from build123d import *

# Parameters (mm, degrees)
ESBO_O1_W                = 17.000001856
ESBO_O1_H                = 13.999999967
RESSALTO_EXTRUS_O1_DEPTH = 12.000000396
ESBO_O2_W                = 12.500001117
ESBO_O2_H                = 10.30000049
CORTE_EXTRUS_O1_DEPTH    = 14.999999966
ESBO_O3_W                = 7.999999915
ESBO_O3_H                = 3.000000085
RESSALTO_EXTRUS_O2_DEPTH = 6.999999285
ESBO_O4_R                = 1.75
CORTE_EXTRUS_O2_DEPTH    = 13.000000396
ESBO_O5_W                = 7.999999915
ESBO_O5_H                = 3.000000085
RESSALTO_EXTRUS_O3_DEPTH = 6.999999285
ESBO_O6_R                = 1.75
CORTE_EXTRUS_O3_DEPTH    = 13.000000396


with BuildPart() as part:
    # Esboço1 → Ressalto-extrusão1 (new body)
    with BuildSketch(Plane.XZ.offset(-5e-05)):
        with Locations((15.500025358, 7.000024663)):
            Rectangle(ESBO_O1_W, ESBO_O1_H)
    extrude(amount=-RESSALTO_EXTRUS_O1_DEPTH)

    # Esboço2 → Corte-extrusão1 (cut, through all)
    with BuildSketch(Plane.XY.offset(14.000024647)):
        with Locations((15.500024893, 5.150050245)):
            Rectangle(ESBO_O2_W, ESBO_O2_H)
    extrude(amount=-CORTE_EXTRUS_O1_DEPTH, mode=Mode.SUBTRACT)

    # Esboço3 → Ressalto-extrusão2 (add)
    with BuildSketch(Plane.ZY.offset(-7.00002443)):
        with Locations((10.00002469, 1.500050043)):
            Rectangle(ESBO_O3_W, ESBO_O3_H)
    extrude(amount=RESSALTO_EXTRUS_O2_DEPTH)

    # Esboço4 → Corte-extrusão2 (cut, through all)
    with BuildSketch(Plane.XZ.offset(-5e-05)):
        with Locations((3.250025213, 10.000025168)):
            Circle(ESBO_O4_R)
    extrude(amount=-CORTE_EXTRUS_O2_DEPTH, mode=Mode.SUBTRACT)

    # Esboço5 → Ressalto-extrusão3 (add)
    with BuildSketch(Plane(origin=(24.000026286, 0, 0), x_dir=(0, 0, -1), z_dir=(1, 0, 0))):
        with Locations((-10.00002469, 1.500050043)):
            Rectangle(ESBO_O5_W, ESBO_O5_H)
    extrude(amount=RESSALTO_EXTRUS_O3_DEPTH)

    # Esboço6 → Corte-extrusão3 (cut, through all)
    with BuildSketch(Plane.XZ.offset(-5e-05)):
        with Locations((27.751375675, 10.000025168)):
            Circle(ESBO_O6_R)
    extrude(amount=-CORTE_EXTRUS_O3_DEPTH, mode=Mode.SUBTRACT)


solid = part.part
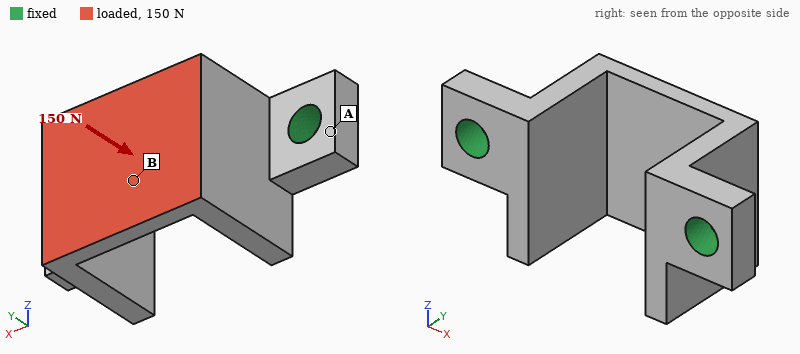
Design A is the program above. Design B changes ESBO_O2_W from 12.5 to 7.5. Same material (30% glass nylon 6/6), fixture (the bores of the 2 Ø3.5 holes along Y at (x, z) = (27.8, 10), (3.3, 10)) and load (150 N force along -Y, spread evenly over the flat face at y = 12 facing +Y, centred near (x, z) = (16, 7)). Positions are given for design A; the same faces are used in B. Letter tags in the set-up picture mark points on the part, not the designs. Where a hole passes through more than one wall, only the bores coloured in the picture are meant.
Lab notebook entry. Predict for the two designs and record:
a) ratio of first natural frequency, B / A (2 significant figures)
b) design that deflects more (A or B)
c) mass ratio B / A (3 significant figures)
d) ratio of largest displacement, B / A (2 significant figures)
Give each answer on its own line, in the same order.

0.86
A
1.54
0.71
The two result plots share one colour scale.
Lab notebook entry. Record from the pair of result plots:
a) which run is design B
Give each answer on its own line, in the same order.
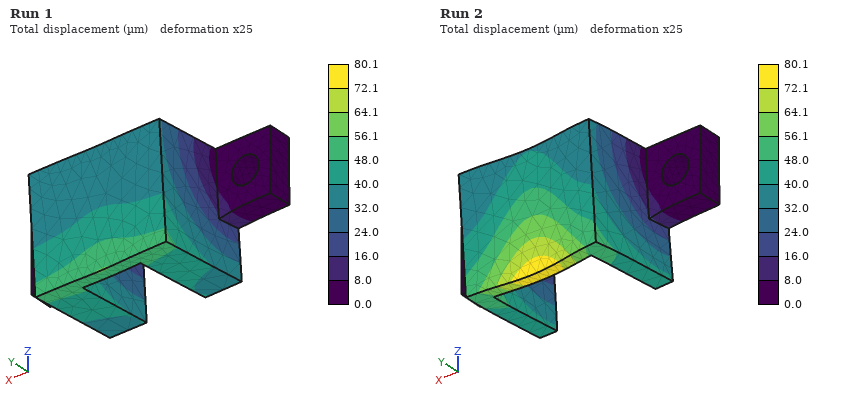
Run 1
